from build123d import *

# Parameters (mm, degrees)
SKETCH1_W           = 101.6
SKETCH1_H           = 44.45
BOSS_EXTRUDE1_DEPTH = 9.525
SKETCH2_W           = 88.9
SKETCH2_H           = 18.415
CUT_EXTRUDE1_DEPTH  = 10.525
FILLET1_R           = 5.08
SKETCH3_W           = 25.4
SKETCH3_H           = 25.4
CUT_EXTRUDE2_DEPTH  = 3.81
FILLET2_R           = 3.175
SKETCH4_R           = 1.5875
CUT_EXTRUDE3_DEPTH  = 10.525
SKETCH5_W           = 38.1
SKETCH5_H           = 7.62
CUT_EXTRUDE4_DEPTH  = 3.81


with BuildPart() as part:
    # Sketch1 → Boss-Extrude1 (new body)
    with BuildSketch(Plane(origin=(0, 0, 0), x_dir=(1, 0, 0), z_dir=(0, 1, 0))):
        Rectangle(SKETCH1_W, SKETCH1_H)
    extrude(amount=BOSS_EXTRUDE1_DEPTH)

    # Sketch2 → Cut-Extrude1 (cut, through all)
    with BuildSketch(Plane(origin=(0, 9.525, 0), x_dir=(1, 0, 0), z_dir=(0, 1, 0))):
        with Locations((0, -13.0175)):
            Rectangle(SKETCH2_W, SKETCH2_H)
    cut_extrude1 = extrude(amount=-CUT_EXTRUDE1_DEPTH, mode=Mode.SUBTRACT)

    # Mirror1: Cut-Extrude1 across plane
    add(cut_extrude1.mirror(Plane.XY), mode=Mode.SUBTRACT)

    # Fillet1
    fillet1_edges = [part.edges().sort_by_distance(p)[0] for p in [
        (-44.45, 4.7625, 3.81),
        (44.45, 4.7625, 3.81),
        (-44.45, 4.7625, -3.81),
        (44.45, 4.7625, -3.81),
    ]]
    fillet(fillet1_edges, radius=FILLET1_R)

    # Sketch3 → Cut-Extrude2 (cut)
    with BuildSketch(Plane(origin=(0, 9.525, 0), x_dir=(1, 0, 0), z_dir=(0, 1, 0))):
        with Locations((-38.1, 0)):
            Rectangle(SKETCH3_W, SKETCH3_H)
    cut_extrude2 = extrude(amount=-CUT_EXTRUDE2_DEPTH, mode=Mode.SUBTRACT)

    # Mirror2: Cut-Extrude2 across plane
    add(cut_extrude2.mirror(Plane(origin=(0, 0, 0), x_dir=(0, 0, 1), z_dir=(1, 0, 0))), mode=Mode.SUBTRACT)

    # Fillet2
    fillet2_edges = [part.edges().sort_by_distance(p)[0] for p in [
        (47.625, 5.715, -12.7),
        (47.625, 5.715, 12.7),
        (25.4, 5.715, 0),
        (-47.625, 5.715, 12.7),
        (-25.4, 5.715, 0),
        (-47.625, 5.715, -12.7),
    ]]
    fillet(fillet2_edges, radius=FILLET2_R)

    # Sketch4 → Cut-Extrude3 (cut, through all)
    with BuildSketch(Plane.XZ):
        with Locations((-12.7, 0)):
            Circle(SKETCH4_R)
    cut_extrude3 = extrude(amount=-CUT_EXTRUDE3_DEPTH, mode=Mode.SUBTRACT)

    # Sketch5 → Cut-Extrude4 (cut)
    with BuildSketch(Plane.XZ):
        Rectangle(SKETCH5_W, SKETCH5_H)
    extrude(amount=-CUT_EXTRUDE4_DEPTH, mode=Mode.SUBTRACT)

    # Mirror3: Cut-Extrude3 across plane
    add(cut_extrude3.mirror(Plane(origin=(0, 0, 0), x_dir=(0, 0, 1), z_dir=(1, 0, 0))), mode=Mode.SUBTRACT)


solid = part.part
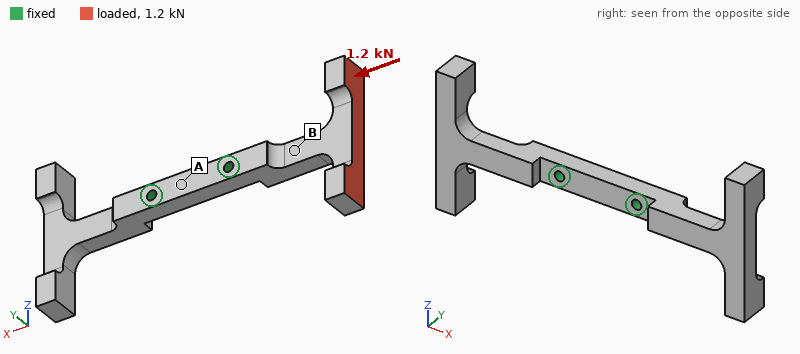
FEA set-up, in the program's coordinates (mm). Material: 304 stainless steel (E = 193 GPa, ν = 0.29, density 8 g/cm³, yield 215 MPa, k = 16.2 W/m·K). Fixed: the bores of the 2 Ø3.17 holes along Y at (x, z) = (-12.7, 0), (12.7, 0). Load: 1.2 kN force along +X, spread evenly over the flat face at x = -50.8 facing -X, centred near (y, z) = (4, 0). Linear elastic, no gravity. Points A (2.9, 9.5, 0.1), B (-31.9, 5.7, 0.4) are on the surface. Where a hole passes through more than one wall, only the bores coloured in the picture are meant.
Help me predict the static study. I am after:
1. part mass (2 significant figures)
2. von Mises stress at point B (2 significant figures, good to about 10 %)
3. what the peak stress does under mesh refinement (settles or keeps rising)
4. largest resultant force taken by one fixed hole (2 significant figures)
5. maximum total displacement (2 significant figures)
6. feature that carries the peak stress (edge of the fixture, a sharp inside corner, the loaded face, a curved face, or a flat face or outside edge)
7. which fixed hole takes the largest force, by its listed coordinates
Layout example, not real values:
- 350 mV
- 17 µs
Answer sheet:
- 68 g
- 60 MPa
- keeps rising
- 1.2 kN
- 41 µm
- edge of the fixture
- (-12.7, 0)
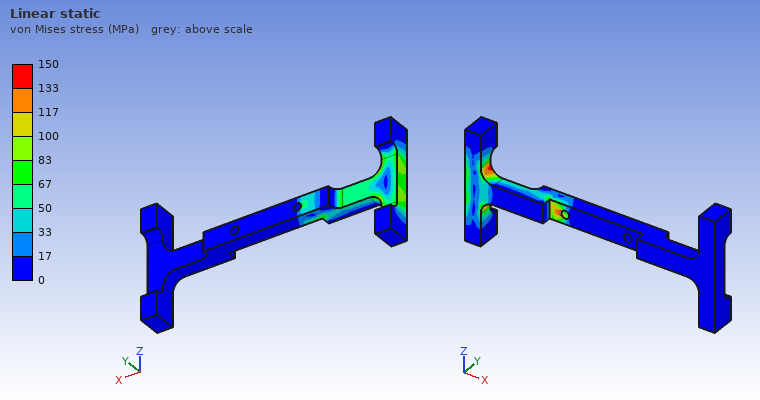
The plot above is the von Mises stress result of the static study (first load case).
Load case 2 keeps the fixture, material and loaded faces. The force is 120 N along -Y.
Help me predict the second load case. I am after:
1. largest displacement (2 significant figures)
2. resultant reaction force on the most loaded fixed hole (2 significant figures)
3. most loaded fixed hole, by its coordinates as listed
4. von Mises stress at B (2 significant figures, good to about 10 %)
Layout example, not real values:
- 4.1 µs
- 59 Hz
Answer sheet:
- 87 µm
- 130 N
- (-12.7, 0)
- 55 MPa
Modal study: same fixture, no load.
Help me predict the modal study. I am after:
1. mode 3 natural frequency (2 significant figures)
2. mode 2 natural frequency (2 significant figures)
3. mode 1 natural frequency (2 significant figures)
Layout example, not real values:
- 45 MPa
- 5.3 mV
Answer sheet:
- 1600 Hz
- 1600 Hz
- 1600 Hz
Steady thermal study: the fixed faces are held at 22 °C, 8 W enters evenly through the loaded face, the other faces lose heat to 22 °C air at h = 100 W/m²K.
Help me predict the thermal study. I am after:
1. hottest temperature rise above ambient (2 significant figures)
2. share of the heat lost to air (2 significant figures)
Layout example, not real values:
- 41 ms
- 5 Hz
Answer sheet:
- 66 K
- 92 %
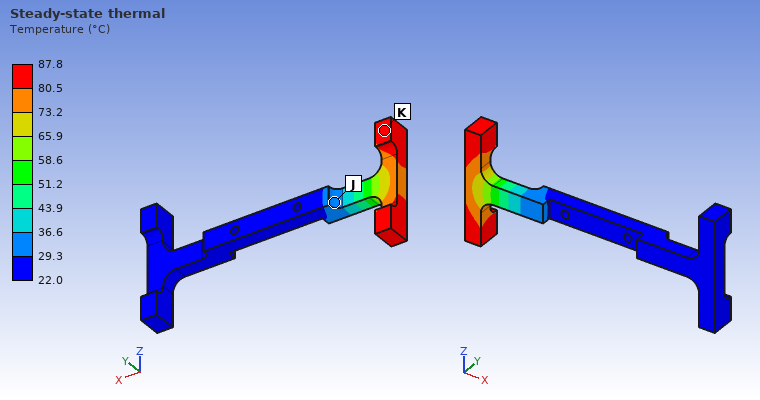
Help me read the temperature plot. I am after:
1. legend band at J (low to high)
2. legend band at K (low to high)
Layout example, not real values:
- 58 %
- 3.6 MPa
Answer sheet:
- 29.3 to 36.6 °C
- 80.5 to 87.8 °C
